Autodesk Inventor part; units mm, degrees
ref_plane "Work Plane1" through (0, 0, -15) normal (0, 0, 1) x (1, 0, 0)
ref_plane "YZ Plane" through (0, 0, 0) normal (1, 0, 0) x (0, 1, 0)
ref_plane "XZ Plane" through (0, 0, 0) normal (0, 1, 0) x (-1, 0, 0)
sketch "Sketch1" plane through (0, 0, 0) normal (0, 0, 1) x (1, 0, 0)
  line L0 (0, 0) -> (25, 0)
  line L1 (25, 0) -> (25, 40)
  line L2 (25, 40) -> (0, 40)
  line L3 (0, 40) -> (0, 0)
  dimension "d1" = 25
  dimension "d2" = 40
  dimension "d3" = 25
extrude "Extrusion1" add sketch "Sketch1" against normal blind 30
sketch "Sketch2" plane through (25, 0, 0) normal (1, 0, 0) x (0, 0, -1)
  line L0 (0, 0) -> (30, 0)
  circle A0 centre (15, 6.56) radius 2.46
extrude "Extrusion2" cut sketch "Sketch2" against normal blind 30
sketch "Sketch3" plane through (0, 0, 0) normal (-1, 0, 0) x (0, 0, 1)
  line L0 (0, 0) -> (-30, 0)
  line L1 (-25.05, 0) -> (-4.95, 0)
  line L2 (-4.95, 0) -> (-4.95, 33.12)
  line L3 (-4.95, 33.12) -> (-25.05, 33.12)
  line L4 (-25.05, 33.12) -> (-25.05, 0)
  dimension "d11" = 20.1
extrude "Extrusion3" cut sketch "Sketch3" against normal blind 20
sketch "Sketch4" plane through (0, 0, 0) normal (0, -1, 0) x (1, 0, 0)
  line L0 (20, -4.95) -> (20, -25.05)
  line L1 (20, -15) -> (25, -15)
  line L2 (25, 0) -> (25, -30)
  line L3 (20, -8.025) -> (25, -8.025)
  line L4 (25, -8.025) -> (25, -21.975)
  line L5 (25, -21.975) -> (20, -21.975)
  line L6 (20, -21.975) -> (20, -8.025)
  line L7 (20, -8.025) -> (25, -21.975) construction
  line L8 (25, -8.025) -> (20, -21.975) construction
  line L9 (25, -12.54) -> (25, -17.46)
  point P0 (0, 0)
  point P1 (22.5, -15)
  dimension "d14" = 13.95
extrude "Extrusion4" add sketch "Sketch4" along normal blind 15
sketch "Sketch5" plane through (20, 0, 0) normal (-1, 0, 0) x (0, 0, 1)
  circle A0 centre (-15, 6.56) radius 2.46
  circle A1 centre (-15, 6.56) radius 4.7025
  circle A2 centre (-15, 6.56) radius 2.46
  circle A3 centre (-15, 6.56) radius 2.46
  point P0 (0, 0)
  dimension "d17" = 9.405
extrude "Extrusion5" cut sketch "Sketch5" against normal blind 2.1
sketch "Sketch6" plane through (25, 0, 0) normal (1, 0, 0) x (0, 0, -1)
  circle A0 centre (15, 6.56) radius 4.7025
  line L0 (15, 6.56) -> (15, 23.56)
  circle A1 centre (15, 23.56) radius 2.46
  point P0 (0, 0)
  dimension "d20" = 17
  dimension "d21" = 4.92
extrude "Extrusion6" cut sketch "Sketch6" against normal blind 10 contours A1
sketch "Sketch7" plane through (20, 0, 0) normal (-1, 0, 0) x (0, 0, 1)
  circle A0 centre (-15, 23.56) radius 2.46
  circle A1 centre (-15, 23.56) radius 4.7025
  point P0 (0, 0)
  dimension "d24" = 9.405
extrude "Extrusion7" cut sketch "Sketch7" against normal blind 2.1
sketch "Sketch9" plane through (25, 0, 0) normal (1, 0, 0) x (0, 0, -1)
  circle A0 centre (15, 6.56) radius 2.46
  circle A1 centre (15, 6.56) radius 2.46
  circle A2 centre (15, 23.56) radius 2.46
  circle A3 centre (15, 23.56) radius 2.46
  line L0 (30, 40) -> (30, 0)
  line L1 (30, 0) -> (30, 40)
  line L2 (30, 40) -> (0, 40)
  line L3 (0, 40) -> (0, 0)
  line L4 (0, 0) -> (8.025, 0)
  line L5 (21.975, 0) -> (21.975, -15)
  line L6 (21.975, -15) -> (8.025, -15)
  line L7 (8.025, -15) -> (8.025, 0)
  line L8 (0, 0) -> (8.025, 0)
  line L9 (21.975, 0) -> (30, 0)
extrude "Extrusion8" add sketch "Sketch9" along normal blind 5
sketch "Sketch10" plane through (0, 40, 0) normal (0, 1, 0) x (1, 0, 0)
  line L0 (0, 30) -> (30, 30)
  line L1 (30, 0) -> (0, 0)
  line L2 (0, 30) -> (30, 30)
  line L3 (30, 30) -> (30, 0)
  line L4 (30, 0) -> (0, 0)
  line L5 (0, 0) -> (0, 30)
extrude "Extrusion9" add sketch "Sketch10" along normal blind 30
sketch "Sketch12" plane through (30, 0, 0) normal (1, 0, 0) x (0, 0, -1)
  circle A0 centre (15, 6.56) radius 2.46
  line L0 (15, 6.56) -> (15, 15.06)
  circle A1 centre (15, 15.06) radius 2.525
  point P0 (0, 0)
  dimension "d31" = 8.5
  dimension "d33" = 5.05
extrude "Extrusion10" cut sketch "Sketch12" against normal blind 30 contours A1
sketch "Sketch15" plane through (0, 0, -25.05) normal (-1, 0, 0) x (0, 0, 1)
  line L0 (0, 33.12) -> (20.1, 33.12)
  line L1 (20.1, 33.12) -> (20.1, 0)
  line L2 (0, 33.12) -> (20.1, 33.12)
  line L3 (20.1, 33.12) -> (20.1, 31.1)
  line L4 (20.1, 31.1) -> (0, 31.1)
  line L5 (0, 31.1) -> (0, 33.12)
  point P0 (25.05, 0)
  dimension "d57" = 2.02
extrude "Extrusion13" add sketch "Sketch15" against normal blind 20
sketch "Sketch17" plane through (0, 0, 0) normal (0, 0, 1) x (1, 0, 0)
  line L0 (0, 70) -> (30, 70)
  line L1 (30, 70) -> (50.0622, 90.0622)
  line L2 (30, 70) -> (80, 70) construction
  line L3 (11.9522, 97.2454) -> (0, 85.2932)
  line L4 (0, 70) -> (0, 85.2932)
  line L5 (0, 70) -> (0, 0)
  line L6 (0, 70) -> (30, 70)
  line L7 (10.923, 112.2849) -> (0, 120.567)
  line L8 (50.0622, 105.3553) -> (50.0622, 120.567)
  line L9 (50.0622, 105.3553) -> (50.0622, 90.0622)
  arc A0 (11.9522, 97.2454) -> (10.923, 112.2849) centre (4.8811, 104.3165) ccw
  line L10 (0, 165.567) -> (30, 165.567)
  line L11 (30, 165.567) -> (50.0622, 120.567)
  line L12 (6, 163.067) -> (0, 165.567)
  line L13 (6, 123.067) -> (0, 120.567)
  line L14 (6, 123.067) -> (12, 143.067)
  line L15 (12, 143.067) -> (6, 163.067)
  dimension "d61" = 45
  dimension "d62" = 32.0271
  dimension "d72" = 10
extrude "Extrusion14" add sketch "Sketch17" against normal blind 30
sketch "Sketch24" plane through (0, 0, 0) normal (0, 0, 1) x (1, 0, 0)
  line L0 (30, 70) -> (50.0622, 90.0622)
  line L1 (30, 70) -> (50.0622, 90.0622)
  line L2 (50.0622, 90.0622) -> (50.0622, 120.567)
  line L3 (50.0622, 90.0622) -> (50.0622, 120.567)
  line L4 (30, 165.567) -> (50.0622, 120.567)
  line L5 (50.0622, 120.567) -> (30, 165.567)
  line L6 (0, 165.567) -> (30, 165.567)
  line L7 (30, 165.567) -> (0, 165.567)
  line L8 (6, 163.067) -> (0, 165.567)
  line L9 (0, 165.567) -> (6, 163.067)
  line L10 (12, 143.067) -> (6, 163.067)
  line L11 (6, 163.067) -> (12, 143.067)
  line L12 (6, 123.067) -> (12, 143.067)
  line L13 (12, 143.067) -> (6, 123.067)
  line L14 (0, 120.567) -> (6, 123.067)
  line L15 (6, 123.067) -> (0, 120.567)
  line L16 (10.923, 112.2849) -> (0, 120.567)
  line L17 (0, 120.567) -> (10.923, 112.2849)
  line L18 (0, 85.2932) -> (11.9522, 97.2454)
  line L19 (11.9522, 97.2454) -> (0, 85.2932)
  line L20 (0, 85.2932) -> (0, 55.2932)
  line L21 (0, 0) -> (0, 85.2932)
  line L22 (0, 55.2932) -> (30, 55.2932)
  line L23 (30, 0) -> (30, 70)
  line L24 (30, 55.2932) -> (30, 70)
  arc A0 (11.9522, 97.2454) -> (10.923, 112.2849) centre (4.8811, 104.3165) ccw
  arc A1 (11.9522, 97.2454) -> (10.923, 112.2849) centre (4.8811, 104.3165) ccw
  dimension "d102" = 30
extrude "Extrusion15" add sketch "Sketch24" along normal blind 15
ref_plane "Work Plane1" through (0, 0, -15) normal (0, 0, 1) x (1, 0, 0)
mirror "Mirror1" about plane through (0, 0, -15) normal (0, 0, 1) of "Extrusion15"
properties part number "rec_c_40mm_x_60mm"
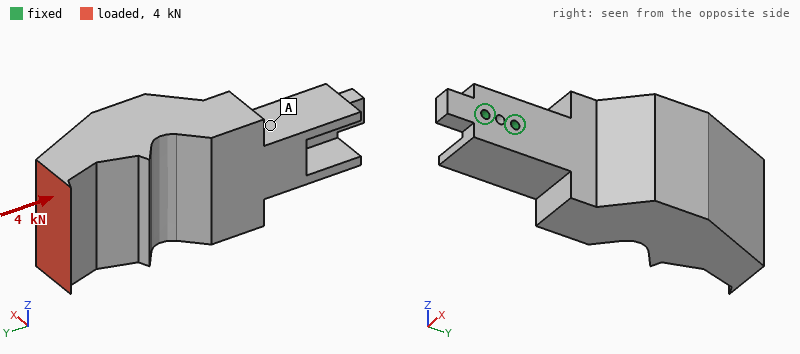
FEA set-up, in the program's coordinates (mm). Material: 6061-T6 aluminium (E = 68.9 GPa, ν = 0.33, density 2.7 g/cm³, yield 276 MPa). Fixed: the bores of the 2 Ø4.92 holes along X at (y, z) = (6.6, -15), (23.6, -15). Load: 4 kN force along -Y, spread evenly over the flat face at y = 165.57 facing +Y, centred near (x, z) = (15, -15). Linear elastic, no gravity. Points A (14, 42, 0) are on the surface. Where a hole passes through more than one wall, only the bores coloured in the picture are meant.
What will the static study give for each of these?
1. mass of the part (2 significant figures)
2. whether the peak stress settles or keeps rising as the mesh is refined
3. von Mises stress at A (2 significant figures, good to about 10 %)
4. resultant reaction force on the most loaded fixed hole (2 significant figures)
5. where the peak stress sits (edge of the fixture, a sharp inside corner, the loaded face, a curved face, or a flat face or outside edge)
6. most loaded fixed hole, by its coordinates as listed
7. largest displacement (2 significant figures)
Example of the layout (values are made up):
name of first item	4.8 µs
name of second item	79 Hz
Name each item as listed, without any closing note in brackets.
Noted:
mass of the part	730 g
whether the peak stress settles or keeps rising as the mesh is refined	keeps rising
von Mises stress at A	6.2 MPa
resultant reaction force on the most loaded fixed hole	3.0 kN
where the peak stress sits	edge of the fixture
most loaded fixed hole, by its coordinates as listed	(23.6, -15)
largest displacement	0.16 mm
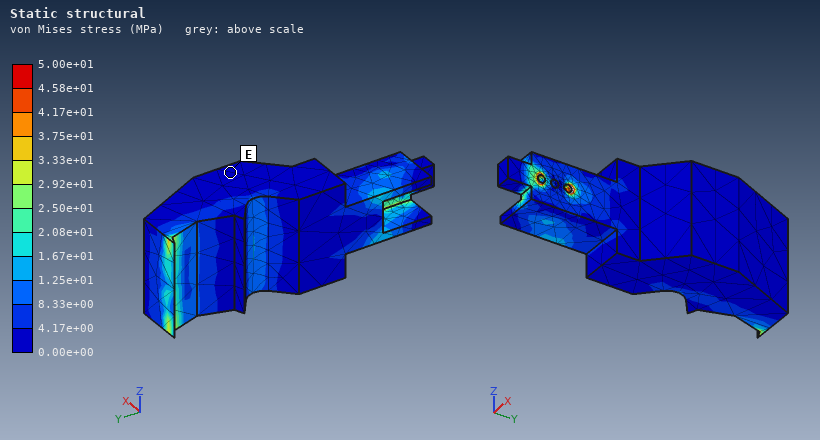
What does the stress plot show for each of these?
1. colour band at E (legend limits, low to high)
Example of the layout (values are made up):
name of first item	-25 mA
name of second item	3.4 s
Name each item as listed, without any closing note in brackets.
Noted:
colour band at E	0.00e+00 to 4.17e+00 MPa
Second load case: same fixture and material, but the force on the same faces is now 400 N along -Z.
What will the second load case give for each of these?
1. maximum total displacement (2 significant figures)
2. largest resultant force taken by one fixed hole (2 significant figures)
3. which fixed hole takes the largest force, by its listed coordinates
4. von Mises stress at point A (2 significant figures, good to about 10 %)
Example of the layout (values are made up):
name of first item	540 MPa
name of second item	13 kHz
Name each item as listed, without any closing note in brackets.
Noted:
maximum total displacement	0.17 mm
largest resultant force taken by one fixed hole	2.9 kN
which fixed hole takes the largest force, by its listed coordinates	(23.6, -15)
von Mises stress at point A	12 MPa
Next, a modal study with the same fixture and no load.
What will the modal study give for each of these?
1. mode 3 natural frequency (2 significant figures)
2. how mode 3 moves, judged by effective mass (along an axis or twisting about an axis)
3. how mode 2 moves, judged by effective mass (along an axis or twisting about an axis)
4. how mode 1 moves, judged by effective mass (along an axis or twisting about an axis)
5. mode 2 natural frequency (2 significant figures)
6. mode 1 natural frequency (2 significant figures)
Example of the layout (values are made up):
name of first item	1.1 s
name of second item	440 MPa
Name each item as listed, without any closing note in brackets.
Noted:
mode 3 natural frequency	1200 Hz
how mode 3 moves, judged by effective mass	twisting about Y
how mode 2 moves, judged by effective mass	along Z
how mode 1 moves, judged by effective mass	along X
mode 2 natural frequency	480 Hz
mode 1 natural frequency	420 Hz
